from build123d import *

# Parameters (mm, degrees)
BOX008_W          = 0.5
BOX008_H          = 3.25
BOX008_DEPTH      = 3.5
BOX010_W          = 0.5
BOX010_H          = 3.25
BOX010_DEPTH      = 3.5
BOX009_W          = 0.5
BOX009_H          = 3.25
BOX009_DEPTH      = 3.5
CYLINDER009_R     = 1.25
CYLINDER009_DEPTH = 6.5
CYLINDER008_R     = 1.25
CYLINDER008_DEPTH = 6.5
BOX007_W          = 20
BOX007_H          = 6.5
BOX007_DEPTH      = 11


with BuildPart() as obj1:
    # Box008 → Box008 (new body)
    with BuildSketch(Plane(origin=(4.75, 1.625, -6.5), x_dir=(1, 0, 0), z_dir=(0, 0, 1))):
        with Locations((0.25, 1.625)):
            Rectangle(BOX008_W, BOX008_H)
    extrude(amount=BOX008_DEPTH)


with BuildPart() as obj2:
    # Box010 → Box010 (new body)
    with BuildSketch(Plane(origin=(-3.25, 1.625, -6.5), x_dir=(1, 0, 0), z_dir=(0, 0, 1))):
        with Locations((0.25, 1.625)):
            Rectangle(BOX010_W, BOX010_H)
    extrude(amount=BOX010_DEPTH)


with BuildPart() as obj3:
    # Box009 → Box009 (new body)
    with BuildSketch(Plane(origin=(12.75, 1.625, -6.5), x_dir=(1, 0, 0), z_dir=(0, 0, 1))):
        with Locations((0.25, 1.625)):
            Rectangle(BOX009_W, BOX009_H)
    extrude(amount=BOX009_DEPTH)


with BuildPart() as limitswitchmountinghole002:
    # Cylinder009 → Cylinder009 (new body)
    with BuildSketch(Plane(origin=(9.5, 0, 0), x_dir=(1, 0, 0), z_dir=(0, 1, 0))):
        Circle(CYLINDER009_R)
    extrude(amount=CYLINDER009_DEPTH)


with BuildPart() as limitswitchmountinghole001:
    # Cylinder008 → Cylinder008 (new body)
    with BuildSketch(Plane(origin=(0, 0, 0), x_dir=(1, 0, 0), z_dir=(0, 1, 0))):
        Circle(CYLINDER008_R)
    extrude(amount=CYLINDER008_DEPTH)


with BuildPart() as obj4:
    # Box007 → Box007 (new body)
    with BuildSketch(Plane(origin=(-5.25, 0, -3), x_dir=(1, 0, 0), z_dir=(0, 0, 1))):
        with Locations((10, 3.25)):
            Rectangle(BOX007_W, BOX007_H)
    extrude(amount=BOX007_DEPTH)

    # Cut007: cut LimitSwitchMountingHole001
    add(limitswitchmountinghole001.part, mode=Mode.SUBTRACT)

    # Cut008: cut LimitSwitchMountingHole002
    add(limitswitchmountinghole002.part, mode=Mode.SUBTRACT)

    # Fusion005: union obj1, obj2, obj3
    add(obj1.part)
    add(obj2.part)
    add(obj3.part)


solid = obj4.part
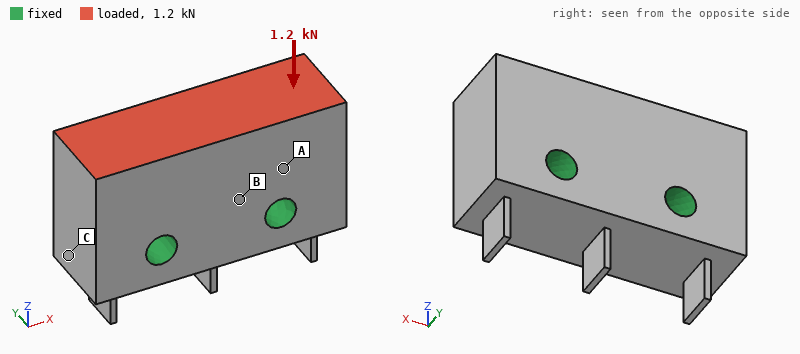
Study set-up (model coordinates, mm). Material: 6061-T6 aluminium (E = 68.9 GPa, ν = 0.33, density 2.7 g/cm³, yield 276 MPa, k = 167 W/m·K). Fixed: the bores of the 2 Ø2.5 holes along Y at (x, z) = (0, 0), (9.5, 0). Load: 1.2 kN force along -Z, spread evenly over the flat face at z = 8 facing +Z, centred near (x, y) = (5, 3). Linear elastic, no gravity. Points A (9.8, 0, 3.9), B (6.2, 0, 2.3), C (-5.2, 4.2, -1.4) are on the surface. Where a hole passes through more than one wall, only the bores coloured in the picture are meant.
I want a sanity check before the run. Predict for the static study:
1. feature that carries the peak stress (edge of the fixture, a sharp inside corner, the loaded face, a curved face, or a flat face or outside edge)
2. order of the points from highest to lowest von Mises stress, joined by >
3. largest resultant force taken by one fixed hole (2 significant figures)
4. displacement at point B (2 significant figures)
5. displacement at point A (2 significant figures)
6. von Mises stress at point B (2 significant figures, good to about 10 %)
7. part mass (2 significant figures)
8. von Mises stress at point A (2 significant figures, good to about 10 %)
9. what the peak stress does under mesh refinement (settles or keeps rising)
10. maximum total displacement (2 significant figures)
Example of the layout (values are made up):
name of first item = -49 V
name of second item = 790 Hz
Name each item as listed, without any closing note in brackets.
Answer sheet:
feature that carries the peak stress = edge of the fixture
order of the points from highest to lowest von Mises stress, joined by > = A > B > C
largest resultant force taken by one fixed hole = 600 N
displacement at point B = 0.52 µm
displacement at point A = 0.67 µm
von Mises stress at point B = 5.4 MPa
part mass = 3.7 g
von Mises stress at point A = 13 MPa
what the peak stress does under mesh refinement = keeps rising
maximum total displacement = 1.8 µm
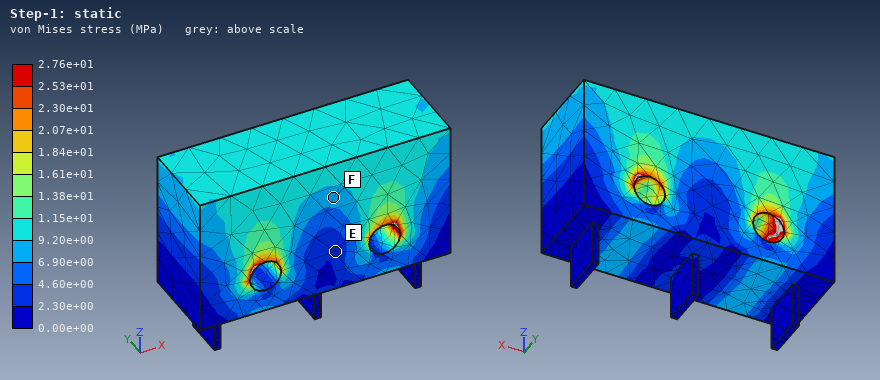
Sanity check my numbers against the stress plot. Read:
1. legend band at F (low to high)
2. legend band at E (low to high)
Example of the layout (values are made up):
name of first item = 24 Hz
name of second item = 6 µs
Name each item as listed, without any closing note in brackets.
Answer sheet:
legend band at F = 6.90e+00 to 9.20e+00 MPa
legend band at E = 2.30e+00 to 4.60e+00 MPa
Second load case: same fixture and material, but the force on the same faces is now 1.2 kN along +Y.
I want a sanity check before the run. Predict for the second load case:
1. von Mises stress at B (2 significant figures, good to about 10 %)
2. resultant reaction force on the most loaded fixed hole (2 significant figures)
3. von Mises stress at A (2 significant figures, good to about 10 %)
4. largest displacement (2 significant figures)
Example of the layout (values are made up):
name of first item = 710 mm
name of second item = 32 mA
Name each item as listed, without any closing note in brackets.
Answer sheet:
von Mises stress at B = 31 MPa
resultant reaction force on the most loaded fixed hole = 600 N
von Mises stress at A = 43 MPa
largest displacement = 12 µm
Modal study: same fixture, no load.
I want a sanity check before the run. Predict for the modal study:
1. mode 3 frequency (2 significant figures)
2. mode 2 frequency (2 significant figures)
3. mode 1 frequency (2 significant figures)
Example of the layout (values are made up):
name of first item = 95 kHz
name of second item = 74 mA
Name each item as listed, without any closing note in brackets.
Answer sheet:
mode 3 frequency = 32 kHz
mode 2 frequency = 32 kHz
mode 1 frequency = 32 kHz
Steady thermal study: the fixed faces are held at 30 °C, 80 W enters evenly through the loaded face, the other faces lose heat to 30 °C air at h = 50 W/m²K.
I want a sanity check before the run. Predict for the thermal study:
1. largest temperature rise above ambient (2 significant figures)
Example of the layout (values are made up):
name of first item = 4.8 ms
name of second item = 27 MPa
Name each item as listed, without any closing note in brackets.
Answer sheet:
largest temperature rise above ambient = 30 K
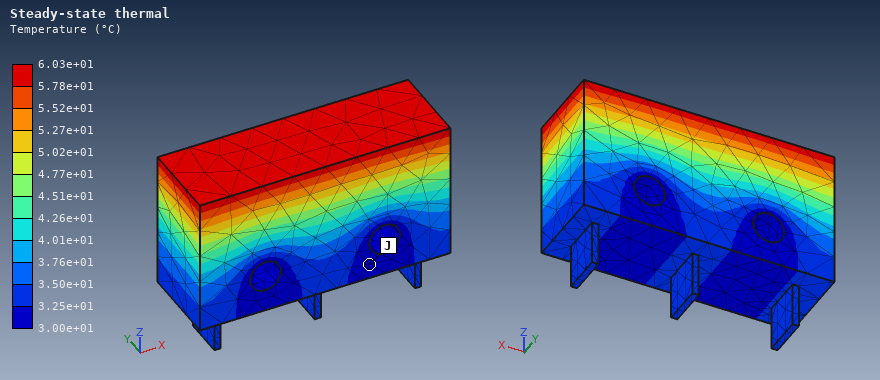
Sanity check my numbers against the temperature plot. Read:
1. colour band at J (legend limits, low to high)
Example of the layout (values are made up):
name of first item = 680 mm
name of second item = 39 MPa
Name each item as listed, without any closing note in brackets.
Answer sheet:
colour band at J = 3.00e+01 to 3.25e+01 °C
